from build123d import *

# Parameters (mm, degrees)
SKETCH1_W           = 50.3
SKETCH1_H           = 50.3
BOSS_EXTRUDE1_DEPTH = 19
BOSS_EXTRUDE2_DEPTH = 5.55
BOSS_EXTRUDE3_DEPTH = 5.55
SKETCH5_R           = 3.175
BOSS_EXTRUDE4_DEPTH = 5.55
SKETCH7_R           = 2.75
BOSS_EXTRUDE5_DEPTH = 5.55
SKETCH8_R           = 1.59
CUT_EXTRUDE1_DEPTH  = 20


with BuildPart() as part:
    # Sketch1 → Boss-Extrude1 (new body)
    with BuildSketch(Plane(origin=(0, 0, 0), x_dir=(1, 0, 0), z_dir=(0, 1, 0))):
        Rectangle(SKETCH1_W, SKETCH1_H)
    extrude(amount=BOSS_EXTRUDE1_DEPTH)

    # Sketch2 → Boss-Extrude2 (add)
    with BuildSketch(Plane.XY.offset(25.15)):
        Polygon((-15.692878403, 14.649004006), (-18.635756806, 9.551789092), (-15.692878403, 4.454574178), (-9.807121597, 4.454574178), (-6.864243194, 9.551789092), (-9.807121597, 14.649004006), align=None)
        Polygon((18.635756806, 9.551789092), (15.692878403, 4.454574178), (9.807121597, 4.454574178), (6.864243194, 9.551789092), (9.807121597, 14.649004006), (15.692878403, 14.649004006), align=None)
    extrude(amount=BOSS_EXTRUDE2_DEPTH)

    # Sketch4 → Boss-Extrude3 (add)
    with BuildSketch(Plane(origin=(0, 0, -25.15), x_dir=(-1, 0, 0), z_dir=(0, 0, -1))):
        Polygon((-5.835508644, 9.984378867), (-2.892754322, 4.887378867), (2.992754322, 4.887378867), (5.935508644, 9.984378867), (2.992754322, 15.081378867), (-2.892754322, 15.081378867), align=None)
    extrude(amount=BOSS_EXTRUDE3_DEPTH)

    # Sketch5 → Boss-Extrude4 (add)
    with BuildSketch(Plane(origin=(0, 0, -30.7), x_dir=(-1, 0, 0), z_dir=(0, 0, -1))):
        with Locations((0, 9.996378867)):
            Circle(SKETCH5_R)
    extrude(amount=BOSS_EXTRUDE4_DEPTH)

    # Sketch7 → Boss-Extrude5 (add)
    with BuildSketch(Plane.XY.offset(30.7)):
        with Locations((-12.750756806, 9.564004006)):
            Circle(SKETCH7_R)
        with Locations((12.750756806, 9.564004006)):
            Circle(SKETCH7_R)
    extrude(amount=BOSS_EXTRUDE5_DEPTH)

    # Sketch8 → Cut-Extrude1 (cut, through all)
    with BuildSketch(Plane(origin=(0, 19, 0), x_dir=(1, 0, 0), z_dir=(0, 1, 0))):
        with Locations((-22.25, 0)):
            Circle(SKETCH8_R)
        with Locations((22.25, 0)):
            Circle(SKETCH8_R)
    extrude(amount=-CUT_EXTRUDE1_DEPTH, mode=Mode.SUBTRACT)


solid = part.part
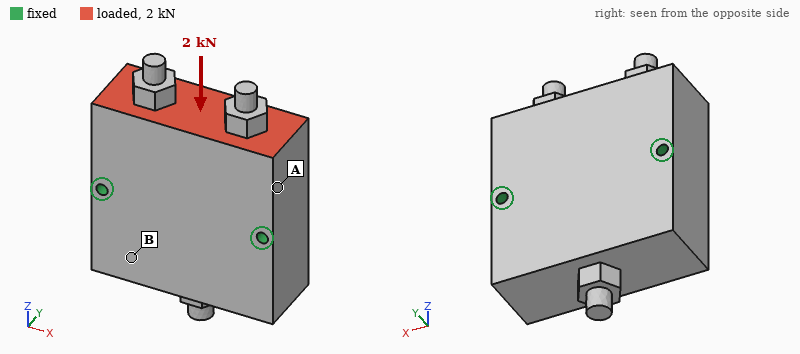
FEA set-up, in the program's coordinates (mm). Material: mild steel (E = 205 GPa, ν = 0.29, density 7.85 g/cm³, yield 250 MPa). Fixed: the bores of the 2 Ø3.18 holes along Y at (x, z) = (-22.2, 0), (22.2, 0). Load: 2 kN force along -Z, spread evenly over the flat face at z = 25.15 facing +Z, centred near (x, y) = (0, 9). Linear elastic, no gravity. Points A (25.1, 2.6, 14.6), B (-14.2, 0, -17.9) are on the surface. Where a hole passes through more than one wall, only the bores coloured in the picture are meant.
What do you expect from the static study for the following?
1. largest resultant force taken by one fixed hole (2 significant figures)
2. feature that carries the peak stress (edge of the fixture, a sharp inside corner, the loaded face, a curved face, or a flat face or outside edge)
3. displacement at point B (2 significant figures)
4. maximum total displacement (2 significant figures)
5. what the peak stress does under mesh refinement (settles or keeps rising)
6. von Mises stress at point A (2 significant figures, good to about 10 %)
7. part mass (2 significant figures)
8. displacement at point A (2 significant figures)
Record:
1.0 kN
edge of the fixture
0.16 µm
0.48 µm
keeps rising
2.9 MPa
390 g
0.25 µm
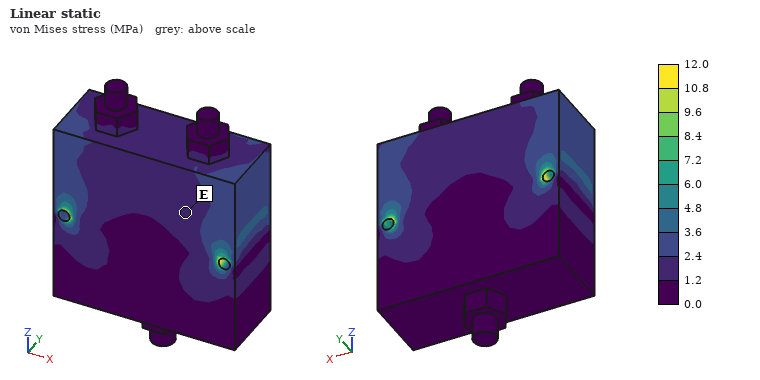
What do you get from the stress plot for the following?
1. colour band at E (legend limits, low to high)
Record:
1.2 to 2.4 MPa
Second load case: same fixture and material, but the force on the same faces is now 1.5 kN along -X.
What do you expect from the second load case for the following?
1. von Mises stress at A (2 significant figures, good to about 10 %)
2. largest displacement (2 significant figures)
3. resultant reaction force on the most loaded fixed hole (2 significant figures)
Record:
2.7 MPa
1.1 µm
1.1 kN
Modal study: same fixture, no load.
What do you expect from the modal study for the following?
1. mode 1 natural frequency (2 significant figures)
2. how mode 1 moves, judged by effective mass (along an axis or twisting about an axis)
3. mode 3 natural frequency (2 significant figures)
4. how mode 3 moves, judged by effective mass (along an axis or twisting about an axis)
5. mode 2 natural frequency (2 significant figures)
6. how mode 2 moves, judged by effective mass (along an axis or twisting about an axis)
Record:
10 kHz
twisting about X
20 kHz
along X
13 kHz
along Y
